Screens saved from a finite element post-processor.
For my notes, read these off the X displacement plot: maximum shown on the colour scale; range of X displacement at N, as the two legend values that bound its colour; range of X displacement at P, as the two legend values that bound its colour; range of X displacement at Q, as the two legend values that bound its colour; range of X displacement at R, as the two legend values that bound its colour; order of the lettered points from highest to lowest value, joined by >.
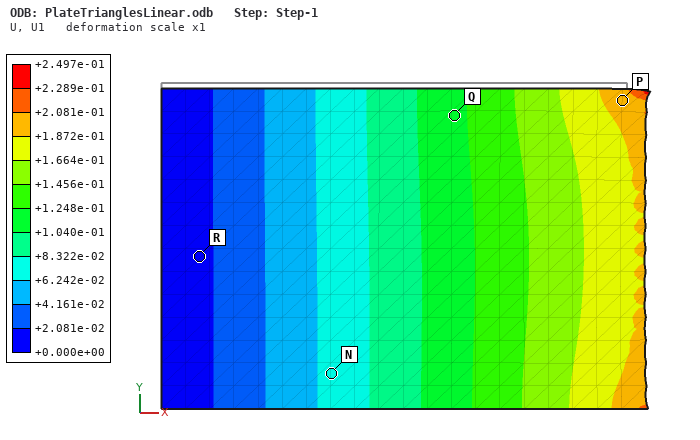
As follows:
+2.497e-01
+6.242e-02 to +8.322e-02
+1.872e-01 to +2.081e-01
+1.040e-01 to +1.248e-01
+0.000e+00 to +2.081e-02
P > Q > N > R
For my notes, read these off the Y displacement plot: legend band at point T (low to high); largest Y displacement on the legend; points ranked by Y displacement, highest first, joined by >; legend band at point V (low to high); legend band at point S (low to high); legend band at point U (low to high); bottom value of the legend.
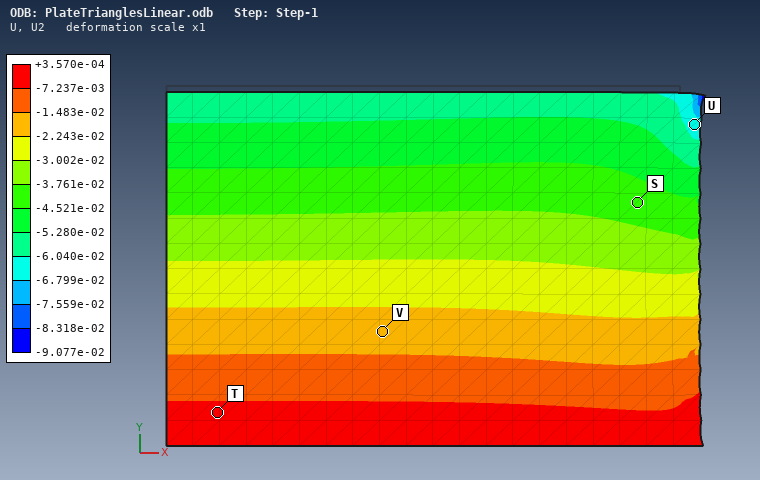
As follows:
-7.237e-03 to +3.570e-04
+3.570e-04
T > V > S > U
-2.243e-02 to -1.483e-02
-4.521e-02 to -3.761e-02
-6.799e-02 to -6.040e-02
-9.077e-02
